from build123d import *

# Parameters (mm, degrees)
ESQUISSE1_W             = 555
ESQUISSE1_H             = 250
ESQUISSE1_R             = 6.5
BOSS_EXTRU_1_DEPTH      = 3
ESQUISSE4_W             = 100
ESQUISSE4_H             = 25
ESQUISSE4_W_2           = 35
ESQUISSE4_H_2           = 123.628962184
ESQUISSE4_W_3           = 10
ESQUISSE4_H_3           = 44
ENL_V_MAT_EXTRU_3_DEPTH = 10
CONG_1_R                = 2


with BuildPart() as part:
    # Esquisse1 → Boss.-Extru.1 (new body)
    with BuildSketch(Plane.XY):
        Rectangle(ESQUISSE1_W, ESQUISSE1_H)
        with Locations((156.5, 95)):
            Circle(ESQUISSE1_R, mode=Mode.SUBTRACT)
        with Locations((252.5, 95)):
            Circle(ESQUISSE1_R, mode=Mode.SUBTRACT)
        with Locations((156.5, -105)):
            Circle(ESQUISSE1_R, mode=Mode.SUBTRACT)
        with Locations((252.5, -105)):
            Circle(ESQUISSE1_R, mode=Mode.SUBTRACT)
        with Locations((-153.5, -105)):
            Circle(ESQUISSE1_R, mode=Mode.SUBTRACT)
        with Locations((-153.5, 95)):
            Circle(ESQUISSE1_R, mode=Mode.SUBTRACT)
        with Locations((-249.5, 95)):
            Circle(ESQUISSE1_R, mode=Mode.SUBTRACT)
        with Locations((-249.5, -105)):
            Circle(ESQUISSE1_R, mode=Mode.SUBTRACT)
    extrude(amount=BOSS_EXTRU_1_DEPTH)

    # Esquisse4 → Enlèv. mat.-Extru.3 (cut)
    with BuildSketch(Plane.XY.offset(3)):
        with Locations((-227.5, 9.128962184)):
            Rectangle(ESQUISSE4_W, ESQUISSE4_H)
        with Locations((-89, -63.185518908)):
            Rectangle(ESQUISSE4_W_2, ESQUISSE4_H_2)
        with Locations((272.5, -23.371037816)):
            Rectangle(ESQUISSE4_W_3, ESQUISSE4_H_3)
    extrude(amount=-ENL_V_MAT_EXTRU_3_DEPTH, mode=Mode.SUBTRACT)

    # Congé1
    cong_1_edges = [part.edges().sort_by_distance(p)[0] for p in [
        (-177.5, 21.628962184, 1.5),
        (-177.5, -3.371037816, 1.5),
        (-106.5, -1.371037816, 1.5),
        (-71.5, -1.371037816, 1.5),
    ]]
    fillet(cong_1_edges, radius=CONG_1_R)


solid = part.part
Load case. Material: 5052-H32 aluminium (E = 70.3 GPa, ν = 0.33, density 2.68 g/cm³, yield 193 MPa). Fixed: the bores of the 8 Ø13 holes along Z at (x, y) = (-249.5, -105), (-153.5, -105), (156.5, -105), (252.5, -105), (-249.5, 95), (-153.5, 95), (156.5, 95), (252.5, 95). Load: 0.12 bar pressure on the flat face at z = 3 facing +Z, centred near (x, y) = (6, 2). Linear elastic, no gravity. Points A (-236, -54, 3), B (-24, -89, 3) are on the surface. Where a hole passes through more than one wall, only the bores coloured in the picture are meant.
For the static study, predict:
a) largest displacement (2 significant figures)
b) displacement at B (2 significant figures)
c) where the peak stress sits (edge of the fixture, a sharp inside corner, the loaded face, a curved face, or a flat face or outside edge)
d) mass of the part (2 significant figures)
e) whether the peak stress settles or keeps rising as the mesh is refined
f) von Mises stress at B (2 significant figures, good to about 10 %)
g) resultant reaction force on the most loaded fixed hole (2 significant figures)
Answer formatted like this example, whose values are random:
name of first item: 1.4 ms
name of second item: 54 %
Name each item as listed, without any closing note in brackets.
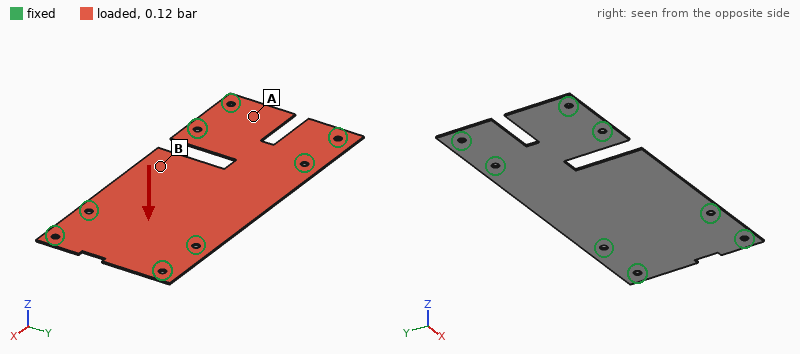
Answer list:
largest displacement: 6.4 mm
displacement at B: 4.8 mm
where the peak stress sits: edge of the fixture
mass of the part: 1.0 kg
whether the peak stress settles or keeps rising as the mesh is refined: keeps rising
von Mises stress at B: 31 MPa
resultant reaction force on the most loaded fixed hole: 370 N
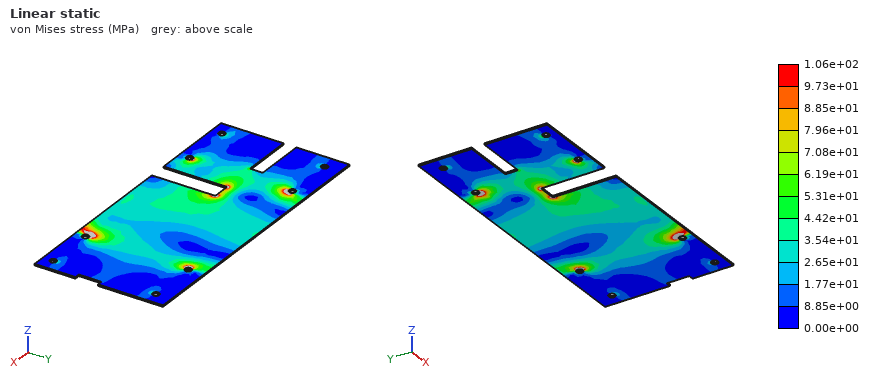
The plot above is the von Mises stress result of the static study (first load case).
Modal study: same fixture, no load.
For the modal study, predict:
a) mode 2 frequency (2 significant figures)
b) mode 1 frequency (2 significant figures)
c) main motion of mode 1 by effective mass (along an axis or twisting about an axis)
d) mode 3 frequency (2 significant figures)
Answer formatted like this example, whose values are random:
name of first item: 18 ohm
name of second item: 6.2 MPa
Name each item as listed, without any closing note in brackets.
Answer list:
mode 2 frequency: 180 Hz
mode 1 frequency: 110 Hz
main motion of mode 1 by effective mass: along Z
mode 3 frequency: 330 Hz
